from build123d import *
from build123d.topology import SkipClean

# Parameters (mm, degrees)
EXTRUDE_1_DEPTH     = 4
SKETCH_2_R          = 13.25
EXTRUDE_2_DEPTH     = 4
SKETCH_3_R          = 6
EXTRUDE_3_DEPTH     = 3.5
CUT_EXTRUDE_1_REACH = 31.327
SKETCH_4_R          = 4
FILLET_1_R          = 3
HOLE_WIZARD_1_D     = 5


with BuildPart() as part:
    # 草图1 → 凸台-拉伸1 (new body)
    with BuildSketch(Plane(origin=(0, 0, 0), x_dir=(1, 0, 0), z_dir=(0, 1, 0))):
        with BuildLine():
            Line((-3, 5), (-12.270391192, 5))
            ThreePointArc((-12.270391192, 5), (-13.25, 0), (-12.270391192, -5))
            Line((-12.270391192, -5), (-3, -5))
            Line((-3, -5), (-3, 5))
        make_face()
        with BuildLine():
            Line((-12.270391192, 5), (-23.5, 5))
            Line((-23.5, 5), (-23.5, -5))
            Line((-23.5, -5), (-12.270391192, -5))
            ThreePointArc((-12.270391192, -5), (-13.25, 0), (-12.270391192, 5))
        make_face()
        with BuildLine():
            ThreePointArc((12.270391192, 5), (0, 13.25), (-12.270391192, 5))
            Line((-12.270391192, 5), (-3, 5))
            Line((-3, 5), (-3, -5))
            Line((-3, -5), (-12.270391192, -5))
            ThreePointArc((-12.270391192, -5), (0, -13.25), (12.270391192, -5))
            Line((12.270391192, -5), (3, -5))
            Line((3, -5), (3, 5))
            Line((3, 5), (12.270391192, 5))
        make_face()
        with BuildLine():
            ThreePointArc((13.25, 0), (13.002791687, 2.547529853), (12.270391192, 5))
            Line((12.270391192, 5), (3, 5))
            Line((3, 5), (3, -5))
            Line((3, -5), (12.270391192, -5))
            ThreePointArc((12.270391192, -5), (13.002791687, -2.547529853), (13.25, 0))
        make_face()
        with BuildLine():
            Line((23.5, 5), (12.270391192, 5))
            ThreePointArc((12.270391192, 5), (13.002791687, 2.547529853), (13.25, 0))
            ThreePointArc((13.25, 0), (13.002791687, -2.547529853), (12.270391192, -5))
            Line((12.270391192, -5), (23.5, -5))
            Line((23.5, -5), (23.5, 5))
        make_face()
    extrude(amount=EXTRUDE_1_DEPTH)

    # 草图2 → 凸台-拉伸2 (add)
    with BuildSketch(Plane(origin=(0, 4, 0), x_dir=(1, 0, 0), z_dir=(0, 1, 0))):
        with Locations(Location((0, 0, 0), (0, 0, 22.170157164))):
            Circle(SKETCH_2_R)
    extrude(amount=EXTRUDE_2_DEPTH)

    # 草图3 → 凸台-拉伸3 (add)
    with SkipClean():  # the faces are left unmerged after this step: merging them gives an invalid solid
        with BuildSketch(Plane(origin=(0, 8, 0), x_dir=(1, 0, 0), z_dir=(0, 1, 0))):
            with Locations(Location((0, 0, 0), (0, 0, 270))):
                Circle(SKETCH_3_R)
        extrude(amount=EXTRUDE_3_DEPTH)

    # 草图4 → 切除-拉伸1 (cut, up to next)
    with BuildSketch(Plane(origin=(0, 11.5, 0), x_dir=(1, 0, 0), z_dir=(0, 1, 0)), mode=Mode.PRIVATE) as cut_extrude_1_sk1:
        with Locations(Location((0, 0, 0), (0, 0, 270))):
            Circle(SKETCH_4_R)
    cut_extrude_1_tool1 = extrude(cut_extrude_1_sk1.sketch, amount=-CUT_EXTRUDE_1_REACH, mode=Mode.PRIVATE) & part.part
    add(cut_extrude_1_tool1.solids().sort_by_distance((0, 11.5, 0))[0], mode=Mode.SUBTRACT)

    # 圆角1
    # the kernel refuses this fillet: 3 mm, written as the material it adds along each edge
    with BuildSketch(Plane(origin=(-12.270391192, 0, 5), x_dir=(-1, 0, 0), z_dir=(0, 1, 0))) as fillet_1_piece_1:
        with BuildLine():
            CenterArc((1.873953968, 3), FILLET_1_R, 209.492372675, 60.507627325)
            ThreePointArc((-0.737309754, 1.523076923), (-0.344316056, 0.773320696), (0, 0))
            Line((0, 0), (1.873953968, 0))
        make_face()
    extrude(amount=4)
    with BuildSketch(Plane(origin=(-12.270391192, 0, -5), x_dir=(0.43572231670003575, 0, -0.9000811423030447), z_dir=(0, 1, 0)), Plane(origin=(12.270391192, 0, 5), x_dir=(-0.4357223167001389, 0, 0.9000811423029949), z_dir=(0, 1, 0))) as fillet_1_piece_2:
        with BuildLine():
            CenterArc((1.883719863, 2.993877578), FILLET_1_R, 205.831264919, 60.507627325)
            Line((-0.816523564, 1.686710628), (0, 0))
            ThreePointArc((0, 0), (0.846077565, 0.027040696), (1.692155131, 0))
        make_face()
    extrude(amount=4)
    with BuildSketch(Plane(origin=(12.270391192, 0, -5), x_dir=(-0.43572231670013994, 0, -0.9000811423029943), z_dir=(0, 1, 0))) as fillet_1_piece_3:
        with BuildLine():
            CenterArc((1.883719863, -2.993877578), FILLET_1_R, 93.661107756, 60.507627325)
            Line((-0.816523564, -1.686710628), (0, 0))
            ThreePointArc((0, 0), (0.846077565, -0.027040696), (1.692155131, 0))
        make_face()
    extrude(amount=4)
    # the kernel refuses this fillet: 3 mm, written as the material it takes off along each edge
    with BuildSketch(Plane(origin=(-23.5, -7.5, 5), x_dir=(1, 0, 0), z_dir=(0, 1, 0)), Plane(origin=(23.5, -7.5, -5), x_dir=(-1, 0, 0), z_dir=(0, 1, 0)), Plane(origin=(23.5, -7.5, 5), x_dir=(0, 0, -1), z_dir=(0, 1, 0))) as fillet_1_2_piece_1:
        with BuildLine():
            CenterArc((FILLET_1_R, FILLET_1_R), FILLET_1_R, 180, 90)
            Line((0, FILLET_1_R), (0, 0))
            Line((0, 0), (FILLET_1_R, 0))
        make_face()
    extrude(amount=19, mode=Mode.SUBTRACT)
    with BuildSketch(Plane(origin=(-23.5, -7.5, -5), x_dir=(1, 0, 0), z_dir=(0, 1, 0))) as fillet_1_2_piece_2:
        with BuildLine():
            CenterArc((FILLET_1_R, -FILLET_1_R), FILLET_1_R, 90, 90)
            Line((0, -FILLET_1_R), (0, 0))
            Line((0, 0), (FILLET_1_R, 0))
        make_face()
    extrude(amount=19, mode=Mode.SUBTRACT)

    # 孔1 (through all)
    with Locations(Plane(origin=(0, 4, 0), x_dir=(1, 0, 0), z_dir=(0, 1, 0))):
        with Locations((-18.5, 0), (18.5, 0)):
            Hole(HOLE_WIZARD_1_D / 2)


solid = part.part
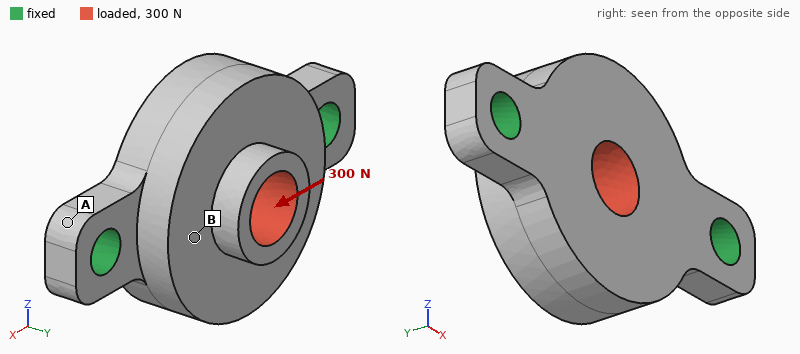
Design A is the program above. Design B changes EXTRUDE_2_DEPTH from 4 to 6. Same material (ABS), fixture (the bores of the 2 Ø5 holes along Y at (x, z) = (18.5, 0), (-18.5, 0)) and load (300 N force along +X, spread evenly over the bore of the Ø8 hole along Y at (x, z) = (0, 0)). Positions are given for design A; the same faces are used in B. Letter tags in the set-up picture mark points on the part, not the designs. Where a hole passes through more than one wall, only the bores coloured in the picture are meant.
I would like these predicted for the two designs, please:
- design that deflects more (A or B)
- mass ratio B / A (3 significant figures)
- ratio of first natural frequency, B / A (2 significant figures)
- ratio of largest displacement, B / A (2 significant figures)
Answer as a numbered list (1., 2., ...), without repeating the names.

1. A
2. 1.18
3. 0.87
4. 0.75
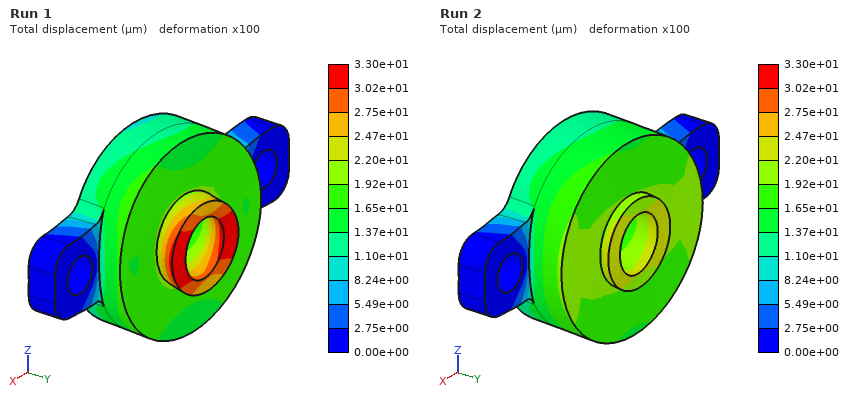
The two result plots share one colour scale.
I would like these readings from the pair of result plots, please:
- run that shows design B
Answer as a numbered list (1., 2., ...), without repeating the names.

1. Run 2
